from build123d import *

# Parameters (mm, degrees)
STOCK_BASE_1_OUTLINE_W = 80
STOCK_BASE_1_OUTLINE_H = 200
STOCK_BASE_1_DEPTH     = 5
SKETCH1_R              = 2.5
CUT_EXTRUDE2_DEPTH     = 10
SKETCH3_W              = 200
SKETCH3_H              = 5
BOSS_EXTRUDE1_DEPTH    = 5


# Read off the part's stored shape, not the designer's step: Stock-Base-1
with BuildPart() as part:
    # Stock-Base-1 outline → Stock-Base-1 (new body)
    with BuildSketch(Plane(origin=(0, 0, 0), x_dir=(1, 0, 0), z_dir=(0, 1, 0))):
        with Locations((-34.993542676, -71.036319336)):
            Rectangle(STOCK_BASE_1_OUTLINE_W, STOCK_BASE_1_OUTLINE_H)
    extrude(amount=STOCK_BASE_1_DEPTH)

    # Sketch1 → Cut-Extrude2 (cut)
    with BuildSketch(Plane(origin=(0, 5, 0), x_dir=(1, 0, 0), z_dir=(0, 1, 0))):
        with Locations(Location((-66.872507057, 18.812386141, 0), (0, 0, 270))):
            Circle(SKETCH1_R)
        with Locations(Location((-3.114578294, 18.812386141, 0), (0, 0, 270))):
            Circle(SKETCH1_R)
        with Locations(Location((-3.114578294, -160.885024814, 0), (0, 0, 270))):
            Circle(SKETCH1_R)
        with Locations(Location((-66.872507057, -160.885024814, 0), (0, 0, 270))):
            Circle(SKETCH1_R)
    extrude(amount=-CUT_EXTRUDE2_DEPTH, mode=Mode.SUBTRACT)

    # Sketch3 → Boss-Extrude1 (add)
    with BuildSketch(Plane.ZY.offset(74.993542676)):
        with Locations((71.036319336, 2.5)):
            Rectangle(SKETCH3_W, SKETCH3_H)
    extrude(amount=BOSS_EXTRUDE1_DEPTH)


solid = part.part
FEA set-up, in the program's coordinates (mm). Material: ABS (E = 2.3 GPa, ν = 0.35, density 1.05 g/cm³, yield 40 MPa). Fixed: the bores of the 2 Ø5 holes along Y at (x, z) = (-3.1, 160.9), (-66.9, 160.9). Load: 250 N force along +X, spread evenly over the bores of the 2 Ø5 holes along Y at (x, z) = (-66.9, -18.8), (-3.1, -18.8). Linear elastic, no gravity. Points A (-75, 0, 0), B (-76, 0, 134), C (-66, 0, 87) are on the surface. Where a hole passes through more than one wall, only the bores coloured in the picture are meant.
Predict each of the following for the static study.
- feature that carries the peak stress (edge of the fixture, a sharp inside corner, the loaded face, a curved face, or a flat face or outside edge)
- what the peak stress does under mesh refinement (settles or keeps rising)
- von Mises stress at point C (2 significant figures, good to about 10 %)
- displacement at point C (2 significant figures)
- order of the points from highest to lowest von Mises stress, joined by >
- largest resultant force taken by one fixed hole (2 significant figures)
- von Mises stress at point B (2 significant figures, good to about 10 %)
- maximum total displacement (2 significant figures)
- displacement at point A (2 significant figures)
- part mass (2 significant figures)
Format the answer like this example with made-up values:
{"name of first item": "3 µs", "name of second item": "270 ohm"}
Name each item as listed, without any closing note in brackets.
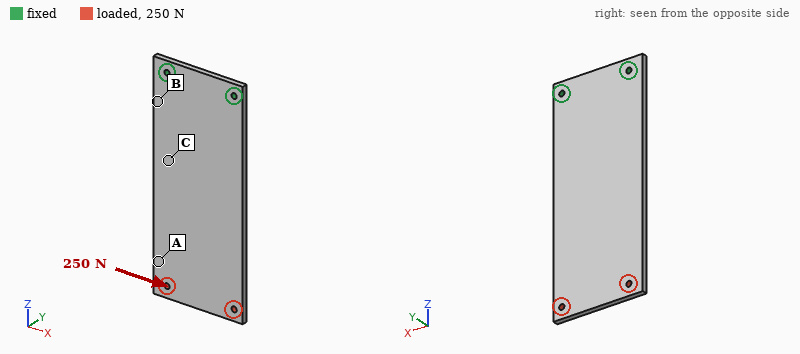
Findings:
{"feature that carries the peak stress": "edge of the fixture", "what the peak stress does under mesh refinement": "keeps rising", "von Mises stress at point C": "3.0 MPa", "displacement at point C": "0.31 mm", "order of the points from highest to lowest von Mises stress, joined by >": "B > C > A", "largest resultant force taken by one fixed hole": "710 N", "von Mises stress at point B": "5.3 MPa", "maximum total displacement": "1.2 mm", "displacement at point A": "0.95 mm", "part mass": "89 g"}
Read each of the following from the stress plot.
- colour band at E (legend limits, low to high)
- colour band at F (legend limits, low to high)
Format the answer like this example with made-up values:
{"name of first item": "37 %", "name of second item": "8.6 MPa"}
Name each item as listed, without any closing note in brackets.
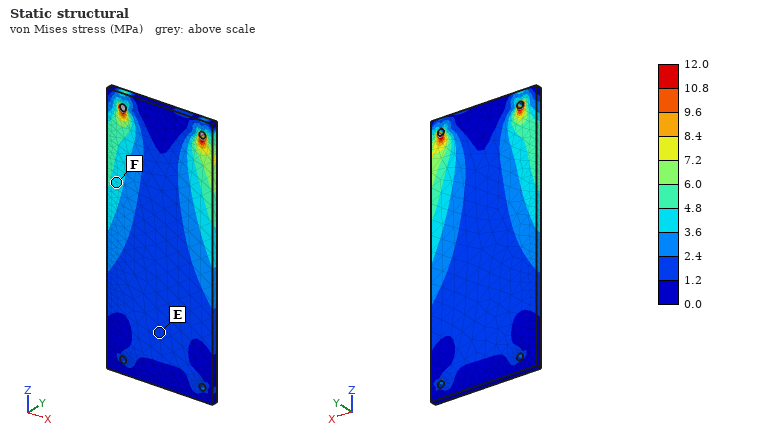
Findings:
{"colour band at E": "1.2 to 2.4 MPa", "colour band at F": "3.6 to 4.8 MPa"}
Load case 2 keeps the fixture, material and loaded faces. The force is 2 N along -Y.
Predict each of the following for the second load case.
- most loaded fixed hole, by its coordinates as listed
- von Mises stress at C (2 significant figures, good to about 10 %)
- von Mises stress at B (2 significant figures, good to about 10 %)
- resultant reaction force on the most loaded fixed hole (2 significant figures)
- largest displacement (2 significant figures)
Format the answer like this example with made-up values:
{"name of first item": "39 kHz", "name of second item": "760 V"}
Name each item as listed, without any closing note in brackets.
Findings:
{"most loaded fixed hole, by its coordinates as listed": "(-66.9, 160.9)", "von Mises stress at C": "0.60 MPa", "von Mises stress at B": "0.94 MPa", "resultant reaction force on the most loaded fixed hole": "1.1 N", "largest displacement": "2.2 mm"}
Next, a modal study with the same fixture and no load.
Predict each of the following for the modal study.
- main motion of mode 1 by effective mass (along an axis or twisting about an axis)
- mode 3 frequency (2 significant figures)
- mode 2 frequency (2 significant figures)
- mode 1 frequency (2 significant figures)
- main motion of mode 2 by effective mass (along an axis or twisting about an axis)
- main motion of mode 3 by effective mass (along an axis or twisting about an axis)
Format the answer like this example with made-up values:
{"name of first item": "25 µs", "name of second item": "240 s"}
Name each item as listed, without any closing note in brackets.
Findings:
{"main motion of mode 1 by effective mass": "along Y", "mode 3 frequency": "200 Hz", "mode 2 frequency": "160 Hz", "mode 1 frequency": "32 Hz", "main motion of mode 2 by effective mass": "twisting about Z", "main motion of mode 3 by effective mass": "along Y"}
